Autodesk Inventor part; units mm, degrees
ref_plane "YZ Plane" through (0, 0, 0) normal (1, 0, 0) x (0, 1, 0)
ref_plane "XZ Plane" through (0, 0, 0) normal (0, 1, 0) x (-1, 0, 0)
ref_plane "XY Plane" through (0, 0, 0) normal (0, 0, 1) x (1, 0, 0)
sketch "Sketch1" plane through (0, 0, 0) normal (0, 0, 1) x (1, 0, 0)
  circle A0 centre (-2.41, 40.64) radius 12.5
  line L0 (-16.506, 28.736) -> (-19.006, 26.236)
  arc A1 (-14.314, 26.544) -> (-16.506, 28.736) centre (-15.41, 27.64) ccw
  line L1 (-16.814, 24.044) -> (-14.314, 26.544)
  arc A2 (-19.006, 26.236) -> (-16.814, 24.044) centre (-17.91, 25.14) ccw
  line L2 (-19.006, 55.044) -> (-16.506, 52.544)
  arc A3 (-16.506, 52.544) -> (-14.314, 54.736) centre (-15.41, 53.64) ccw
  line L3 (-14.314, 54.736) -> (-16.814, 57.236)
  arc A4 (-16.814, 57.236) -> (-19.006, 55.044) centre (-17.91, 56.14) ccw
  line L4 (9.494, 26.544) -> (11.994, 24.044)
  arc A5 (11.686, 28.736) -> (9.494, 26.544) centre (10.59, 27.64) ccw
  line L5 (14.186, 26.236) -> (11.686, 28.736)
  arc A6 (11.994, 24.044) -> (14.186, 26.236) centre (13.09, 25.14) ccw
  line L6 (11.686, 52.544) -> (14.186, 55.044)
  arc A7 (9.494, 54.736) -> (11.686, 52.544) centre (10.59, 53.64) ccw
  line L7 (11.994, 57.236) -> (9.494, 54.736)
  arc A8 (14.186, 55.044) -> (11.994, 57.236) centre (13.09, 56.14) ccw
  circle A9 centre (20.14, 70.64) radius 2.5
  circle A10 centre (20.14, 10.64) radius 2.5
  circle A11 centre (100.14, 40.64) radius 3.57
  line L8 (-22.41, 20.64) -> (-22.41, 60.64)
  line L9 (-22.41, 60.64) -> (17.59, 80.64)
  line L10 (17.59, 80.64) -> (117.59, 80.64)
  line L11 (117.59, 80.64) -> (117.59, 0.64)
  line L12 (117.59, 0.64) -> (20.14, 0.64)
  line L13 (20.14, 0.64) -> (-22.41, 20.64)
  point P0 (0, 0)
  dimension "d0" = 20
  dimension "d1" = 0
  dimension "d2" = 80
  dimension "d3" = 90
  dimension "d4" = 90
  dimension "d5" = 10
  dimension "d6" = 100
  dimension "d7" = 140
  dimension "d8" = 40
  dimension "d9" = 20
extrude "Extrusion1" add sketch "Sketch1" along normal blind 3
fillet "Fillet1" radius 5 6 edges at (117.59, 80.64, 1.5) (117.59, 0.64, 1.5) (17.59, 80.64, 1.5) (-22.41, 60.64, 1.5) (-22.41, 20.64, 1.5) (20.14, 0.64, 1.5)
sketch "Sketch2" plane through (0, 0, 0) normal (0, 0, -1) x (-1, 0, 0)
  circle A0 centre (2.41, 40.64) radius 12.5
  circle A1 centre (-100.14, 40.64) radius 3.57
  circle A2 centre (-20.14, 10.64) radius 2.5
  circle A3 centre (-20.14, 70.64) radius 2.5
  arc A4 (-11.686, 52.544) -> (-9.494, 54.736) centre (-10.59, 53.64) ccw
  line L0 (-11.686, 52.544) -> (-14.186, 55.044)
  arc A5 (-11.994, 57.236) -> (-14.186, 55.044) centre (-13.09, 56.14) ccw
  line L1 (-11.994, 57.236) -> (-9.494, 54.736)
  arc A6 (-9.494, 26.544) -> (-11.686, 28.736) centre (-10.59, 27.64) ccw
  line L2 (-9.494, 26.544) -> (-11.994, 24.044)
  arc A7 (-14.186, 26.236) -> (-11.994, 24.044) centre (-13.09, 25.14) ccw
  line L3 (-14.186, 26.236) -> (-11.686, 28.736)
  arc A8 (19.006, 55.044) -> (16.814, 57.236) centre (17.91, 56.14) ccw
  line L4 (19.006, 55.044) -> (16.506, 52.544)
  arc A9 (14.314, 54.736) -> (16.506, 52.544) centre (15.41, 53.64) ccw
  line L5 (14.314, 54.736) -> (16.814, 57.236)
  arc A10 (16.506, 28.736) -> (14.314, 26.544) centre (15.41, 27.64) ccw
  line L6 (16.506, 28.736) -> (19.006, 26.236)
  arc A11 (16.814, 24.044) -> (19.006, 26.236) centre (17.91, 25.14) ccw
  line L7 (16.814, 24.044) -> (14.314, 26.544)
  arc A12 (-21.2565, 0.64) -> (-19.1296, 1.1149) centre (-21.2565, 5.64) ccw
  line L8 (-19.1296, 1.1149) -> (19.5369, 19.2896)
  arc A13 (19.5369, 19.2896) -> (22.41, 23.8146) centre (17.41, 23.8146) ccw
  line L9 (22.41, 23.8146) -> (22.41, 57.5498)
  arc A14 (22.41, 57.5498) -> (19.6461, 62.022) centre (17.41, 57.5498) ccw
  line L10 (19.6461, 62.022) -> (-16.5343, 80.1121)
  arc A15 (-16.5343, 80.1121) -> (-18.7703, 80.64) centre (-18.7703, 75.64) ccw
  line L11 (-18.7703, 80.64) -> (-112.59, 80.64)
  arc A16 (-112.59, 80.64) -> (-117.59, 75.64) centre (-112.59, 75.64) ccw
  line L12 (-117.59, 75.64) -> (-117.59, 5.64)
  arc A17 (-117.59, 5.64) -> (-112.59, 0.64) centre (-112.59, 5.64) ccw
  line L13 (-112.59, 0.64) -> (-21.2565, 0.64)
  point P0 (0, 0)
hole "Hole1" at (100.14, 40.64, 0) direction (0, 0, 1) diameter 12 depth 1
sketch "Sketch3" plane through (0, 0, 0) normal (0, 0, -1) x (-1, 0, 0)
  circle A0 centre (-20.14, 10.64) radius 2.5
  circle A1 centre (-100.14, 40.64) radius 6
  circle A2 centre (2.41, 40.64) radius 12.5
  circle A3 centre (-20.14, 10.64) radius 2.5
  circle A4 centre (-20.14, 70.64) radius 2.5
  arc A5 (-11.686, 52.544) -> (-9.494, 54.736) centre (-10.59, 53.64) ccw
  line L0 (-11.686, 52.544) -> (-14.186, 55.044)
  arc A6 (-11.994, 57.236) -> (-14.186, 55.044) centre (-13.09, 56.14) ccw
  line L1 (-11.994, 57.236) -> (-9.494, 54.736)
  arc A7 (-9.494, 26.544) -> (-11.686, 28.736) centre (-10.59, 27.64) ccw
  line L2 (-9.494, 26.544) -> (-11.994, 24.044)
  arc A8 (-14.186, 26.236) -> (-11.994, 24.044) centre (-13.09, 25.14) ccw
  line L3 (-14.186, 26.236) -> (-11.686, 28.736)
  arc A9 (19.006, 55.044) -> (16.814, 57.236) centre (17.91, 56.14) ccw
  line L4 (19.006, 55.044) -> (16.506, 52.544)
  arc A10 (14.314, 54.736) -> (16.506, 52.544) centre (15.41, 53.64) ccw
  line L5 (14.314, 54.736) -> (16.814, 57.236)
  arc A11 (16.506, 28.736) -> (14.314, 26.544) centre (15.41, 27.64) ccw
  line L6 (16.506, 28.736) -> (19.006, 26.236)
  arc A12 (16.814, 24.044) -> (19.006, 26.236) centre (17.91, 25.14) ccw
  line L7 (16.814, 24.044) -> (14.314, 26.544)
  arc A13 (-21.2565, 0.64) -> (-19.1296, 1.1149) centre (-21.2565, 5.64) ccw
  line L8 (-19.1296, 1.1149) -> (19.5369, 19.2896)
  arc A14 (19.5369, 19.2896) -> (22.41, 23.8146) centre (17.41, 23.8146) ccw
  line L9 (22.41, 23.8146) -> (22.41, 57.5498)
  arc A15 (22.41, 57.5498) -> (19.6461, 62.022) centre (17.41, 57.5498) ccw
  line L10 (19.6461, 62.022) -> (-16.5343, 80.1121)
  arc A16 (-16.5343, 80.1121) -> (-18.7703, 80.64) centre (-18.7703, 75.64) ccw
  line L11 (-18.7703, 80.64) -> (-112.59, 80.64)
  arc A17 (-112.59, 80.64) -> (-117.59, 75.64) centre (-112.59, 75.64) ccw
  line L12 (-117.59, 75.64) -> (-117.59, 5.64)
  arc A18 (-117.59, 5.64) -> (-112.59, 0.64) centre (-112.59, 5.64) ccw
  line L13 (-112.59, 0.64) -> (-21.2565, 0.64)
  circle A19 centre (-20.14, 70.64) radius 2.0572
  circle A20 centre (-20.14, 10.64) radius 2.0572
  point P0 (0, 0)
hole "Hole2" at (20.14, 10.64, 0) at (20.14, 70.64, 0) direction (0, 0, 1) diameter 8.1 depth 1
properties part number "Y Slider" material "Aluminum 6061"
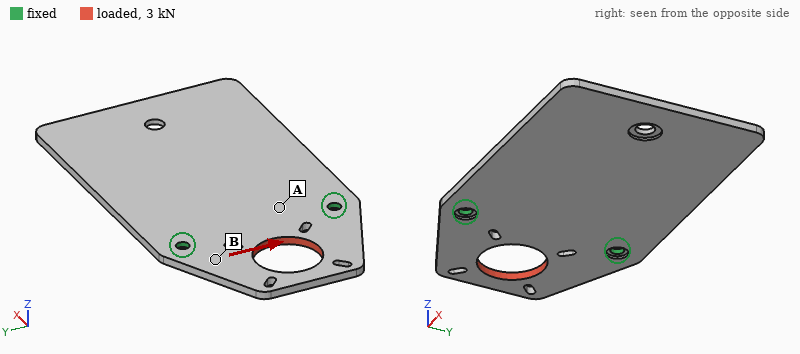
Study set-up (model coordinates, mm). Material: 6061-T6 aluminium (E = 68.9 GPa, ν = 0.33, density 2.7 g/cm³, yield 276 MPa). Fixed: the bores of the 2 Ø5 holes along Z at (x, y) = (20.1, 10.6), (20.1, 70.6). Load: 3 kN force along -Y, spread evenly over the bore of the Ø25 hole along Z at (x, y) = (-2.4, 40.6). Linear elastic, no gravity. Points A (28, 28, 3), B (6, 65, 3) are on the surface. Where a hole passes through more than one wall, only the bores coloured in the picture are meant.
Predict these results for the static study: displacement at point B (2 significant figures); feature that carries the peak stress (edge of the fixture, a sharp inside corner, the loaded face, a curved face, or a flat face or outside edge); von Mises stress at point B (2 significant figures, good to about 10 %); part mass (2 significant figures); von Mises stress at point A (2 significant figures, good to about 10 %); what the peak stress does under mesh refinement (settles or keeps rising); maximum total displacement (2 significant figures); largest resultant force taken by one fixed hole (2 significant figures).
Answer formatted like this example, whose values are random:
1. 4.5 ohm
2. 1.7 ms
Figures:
1. 16 µm
2. edge of the fixture
3. 28 MPa
4. 78 g
5. 11 MPa
6. keeps rising
7. 50 µm
8. 1.9 kN
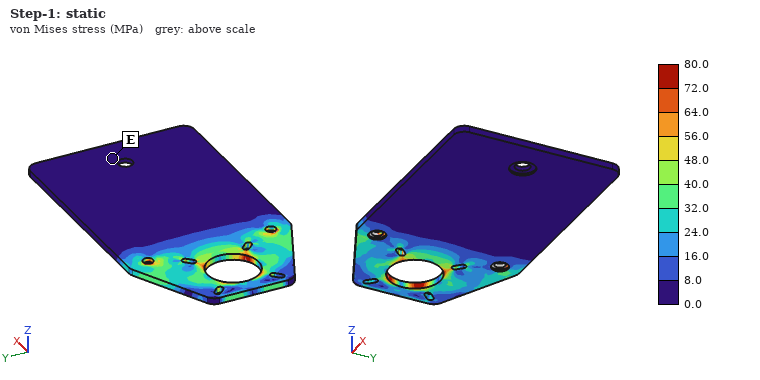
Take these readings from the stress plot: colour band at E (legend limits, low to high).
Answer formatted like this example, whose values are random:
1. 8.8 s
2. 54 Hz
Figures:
1. 0.0 to 8.0 MPa
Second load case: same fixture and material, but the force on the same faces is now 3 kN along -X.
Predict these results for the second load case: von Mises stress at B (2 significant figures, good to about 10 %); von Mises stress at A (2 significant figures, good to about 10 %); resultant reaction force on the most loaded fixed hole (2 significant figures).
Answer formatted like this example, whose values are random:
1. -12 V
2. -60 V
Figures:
1. 21 MPa
2. 9.2 MPa
3. 1.5 kN
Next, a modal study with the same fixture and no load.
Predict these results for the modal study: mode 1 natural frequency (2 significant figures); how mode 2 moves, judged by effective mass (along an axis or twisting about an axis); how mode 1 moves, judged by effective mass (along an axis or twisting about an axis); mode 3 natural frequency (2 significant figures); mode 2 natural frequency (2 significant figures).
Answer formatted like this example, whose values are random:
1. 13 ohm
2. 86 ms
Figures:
1. 230 Hz
2. twisting about X
3. along Z
4. 1300 Hz
5. 730 Hz
